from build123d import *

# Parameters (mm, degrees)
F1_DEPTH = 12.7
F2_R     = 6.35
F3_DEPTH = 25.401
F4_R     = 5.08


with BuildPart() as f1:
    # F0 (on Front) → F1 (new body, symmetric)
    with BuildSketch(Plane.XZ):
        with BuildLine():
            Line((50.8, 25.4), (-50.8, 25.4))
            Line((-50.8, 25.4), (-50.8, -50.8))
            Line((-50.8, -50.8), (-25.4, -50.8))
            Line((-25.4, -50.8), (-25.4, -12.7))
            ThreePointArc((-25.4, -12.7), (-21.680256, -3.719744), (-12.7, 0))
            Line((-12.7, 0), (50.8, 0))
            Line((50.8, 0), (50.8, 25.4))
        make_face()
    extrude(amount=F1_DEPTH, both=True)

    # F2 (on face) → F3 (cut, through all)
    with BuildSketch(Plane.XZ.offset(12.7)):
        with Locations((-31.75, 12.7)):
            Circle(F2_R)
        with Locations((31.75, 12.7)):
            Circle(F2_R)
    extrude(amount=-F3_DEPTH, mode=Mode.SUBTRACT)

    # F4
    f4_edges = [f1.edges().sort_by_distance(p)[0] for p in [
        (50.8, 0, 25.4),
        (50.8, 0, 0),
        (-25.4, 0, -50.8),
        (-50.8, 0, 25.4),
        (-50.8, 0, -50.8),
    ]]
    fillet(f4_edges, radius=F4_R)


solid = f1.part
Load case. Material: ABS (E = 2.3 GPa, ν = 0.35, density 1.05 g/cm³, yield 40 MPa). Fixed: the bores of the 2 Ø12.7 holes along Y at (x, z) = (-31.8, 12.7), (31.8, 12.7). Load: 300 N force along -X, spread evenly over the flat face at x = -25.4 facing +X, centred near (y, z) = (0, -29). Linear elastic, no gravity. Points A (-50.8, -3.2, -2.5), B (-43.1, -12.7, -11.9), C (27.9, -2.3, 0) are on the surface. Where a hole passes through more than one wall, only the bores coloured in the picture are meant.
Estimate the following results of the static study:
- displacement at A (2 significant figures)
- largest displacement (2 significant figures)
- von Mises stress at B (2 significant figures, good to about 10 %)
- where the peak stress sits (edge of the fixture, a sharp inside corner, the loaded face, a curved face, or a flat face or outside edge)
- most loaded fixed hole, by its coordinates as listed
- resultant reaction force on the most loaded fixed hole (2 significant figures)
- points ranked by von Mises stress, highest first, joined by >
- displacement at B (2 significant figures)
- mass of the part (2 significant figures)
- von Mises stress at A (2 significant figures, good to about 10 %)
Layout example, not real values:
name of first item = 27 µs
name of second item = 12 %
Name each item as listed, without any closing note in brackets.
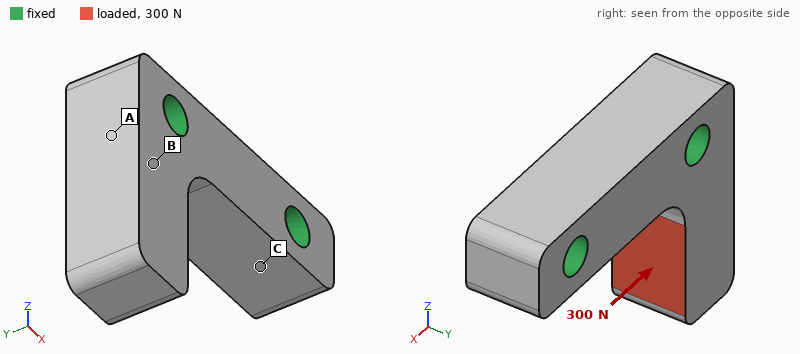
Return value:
displacement at A = 0.035 mm
largest displacement = 0.16 mm
von Mises stress at B = 1.1 MPa
where the peak stress sits = edge of the fixture
most loaded fixed hole, by its coordinates as listed = (-31.8, 12.7)
resultant reaction force on the most loaded fixed hole = 240 N
points ranked by von Mises stress, highest first, joined by > = A > B > C
displacement at B = 0.041 mm
mass of the part = 97 g
von Mises stress at A = 2.1 MPa
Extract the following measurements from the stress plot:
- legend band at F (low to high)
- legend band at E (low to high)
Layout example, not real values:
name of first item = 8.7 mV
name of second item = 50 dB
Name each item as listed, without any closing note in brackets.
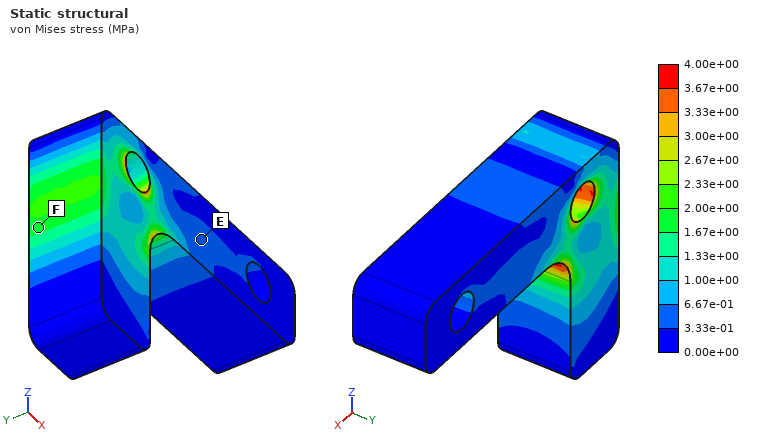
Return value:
legend band at F = 1.67e+00 to 2.00e+00 MPa
legend band at E = 3.33e-01 to 6.67e-01 MPa
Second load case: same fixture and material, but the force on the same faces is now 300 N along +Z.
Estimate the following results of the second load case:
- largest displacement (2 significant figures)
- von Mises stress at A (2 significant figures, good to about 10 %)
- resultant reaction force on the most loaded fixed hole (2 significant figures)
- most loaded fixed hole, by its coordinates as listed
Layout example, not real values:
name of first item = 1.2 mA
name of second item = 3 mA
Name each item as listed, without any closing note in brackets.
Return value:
largest displacement = 59 µm
von Mises stress at A = 0.61 MPa
resultant reaction force on the most loaded fixed hole = 280 N
most loaded fixed hole, by its coordinates as listed = (-31.8, 12.7)
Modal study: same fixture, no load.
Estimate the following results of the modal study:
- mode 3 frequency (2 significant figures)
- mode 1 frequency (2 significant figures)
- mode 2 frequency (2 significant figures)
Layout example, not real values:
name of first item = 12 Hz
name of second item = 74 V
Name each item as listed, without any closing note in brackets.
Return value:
mode 3 frequency = 3700 Hz
mode 1 frequency = 1500 Hz
mode 2 frequency = 1500 Hz
